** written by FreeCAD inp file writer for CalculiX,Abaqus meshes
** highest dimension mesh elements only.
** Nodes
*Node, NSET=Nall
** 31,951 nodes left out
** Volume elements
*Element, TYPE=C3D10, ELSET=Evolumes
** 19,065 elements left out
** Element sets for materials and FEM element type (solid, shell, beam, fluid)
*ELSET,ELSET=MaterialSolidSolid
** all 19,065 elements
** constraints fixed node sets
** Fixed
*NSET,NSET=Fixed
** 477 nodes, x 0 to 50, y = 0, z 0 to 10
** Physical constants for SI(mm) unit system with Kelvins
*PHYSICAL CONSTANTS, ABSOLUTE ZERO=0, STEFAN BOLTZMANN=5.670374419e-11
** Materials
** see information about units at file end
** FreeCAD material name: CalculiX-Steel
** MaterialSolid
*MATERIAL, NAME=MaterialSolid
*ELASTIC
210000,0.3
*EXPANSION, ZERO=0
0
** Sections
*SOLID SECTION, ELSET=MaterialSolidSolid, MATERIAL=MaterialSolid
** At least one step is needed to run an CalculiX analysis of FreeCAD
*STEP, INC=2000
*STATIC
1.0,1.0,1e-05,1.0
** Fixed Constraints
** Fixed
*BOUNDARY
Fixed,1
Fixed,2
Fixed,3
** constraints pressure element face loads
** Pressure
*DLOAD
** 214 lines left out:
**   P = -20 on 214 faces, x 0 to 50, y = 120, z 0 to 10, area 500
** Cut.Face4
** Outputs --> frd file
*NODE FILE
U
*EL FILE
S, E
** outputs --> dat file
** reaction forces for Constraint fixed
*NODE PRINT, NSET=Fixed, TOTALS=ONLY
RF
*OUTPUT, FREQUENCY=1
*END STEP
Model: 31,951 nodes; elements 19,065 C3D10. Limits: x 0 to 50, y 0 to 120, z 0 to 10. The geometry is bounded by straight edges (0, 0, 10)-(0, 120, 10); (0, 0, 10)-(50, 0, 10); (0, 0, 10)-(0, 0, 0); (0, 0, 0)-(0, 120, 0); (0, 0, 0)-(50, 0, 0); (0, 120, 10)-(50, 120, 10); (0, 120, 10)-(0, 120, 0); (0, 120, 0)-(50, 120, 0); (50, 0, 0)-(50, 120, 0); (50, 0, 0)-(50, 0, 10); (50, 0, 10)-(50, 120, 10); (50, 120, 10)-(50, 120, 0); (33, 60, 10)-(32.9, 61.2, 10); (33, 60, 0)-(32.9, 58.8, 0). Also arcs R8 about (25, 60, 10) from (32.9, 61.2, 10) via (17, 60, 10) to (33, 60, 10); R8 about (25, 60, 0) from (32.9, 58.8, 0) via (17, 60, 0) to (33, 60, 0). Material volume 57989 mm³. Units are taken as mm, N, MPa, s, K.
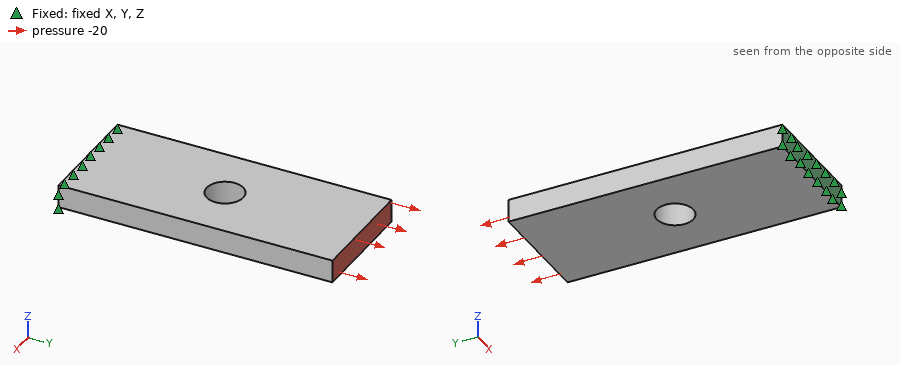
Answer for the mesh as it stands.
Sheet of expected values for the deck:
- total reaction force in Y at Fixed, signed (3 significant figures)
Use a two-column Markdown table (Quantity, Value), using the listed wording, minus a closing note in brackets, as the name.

| Quantity | Value |
|---|---|
| total reaction force in Y at Fixed, signed | -10000 N |
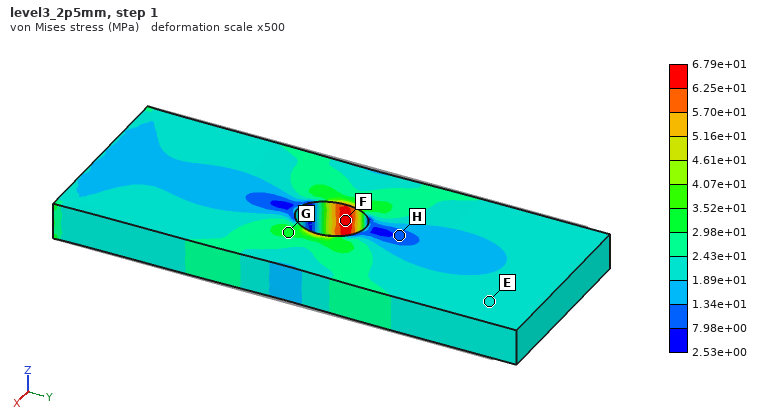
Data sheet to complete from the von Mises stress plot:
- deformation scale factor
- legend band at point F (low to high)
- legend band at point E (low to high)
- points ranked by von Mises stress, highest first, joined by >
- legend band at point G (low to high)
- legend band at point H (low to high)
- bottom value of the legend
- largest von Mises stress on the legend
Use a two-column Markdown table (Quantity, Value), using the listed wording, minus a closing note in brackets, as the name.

| Quantity | Value |
|---|---|
| deformation scale factor | 500 |
| legend band at point F | 6.25e+01 to 6.79e+01 MPa |
| legend band at point E | 1.89e+01 to 2.43e+01 MPa |
| points ranked by von Mises stress, highest first, joined by > | F > G > E > H |
| legend band at point G | 2.98e+01 to 3.52e+01 MPa |
| legend band at point H | 7.98e+00 to 1.34e+01 MPa |
| bottom value of the legend | 2.53e+00 MPa |
| largest von Mises stress on the legend | 6.79e+01 MPa |
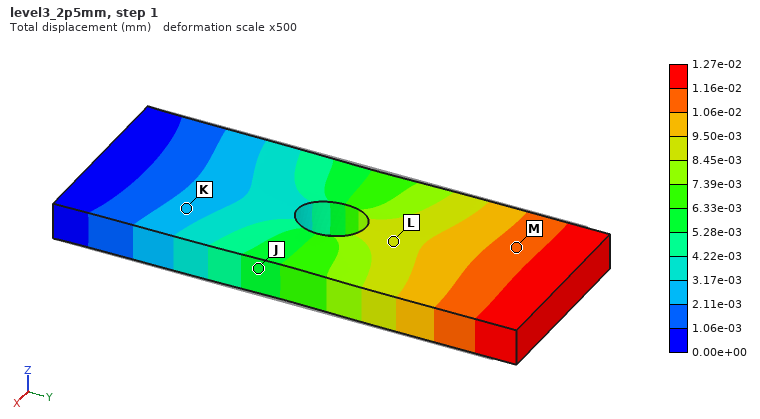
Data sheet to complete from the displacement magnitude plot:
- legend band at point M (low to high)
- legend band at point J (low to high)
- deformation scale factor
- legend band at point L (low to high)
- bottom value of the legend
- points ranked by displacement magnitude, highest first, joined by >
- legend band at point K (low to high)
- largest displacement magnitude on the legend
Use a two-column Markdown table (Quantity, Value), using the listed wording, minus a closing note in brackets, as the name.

| Quantity | Value |
|---|---|
| legend band at point M | 1.06e-02 to 1.16e-02 mm |
| legend band at point J | 5.28e-03 to 6.33e-03 mm |
| deformation scale factor | 500 |
| legend band at point L | 8.45e-03 to 9.50e-03 mm |
| bottom value of the legend | 0.00e+00 mm |
| points ranked by displacement magnitude, highest first, joined by > | M > L > J > K |
| legend band at point K | 2.11e-03 to 3.17e-03 mm |
| largest displacement magnitude on the legend | 1.27e-02 mm |
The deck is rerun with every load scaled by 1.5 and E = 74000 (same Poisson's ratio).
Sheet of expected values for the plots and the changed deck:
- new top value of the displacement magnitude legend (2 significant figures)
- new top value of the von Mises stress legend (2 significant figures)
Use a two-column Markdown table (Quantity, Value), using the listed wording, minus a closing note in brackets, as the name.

| Quantity | Value |
|---|---|
| new top value of the displacement magnitude legend | 0.054 mm |
| new top value of the von Mises stress legend | 100 MPa |
